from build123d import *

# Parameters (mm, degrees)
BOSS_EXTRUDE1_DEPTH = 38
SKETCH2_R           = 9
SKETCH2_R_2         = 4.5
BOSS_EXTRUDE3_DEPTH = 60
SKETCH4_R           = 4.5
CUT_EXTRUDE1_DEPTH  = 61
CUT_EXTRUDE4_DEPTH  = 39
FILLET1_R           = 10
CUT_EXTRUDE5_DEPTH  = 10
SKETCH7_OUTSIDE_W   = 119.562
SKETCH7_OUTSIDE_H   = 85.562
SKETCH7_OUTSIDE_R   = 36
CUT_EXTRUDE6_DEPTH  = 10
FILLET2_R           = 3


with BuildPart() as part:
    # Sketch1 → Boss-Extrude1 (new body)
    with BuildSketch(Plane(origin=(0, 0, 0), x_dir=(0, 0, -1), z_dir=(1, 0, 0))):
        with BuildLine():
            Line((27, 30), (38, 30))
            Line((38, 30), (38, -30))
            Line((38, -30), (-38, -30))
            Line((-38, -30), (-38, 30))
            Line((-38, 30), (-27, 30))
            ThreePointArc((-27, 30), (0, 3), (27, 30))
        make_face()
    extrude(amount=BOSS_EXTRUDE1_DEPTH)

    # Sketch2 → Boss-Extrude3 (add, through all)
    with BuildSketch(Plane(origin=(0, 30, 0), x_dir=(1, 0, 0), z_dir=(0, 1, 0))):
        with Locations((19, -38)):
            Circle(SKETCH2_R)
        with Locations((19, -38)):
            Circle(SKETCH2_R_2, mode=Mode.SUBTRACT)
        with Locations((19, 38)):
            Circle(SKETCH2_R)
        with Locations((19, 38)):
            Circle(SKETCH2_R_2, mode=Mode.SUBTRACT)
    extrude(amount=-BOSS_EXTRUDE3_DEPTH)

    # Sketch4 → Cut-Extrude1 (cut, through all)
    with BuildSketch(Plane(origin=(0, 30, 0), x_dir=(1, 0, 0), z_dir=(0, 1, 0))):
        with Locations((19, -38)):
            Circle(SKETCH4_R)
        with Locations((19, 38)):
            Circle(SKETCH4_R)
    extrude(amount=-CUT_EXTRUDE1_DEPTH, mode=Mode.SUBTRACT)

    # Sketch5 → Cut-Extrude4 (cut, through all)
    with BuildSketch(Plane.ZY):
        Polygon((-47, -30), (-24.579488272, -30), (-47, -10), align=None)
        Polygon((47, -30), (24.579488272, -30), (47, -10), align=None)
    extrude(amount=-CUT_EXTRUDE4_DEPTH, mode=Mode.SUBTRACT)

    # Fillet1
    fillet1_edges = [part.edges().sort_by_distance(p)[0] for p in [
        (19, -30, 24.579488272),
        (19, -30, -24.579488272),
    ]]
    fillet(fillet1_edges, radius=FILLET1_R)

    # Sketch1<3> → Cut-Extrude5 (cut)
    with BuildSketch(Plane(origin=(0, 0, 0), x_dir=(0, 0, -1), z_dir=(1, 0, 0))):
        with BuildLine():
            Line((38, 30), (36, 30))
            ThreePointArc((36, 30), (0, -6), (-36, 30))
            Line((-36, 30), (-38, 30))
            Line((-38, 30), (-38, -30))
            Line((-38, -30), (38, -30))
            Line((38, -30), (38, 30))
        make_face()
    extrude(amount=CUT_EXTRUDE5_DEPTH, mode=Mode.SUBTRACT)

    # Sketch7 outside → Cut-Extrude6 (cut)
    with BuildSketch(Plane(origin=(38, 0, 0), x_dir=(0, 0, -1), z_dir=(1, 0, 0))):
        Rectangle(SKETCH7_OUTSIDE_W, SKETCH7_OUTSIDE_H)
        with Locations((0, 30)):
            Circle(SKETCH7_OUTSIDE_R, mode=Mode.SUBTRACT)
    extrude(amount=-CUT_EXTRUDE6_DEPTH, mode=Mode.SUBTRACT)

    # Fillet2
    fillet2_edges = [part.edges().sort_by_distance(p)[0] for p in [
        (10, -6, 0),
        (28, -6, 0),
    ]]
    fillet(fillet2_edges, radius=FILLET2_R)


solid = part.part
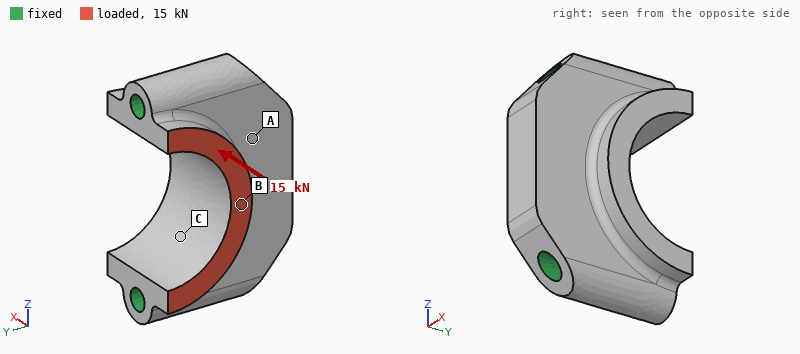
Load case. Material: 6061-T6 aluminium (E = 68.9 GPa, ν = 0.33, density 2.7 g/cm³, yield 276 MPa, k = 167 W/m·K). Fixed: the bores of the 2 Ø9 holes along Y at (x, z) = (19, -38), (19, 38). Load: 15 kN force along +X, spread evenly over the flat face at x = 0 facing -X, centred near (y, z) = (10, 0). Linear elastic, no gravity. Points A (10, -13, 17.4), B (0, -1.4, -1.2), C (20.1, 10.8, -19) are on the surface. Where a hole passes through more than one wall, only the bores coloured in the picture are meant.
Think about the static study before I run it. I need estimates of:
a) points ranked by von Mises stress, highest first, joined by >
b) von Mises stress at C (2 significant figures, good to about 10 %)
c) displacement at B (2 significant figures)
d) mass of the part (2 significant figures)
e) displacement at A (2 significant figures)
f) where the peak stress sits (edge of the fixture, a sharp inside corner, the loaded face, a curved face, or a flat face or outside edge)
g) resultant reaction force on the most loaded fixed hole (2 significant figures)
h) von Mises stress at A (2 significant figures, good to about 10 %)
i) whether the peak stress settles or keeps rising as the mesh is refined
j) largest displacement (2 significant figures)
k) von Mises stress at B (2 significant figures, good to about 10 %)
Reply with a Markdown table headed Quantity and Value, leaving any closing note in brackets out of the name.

| Quantity | Value |
|---|---|
| points ranked by von Mises stress, highest first, joined by > | B > C > A |
| von Mises stress at C | 12 MPa |
| displacement at B | 15 µm |
| mass of the part | 220 g |
| displacement at A | 7.7 µm |
| where the peak stress sits | edge of the fixture |
| resultant reaction force on the most loaded fixed hole | 7.5 kN |
| von Mises stress at A | 5.9 MPa |
| whether the peak stress settles or keeps rising as the mesh is refined | keeps rising |
| largest displacement | 15 µm |
| von Mises stress at B | 20 MPa |
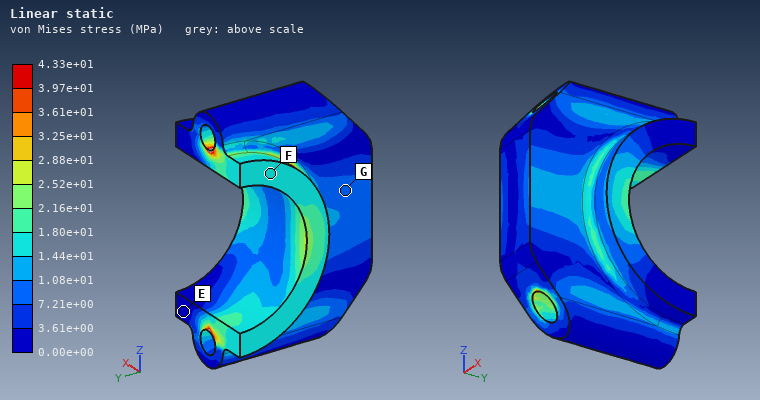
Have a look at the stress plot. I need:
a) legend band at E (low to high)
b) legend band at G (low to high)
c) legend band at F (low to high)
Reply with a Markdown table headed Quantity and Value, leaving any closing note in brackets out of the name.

| Quantity | Value |
|---|---|
| legend band at E | 0.00e+00 to 3.61e+00 MPa |
| legend band at G | 7.21e+00 to 1.08e+01 MPa |
| legend band at F | 1.44e+01 to 1.80e+01 MPa |
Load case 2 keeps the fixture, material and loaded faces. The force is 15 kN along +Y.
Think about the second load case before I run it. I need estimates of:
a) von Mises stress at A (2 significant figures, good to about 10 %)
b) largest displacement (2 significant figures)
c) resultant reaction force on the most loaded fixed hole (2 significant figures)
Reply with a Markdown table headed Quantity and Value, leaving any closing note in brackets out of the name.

| Quantity | Value |
|---|---|
| von Mises stress at A | 16 MPa |
| largest displacement | 41 µm |
| resultant reaction force on the most loaded fixed hole | 7.7 kN |
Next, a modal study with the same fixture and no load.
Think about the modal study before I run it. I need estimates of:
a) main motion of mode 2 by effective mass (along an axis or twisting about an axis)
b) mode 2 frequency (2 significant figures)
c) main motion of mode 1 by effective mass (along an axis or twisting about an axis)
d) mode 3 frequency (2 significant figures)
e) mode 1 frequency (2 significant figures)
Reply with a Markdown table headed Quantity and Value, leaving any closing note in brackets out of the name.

| Quantity | Value |
|---|---|
| main motion of mode 2 by effective mass | along Y |
| mode 2 frequency | 19 kHz |
| main motion of mode 1 by effective mass | along X |
| mode 3 frequency | 20 kHz |
| mode 1 frequency | 12 kHz |
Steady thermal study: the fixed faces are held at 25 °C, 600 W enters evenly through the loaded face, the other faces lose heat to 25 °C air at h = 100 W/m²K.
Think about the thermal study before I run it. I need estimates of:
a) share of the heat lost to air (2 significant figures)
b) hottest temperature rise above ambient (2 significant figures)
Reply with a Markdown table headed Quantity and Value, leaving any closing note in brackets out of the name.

| Quantity | Value |
|---|---|
| share of the heat lost to air | 4.5 % |
| hottest temperature rise above ambient | 84 K |
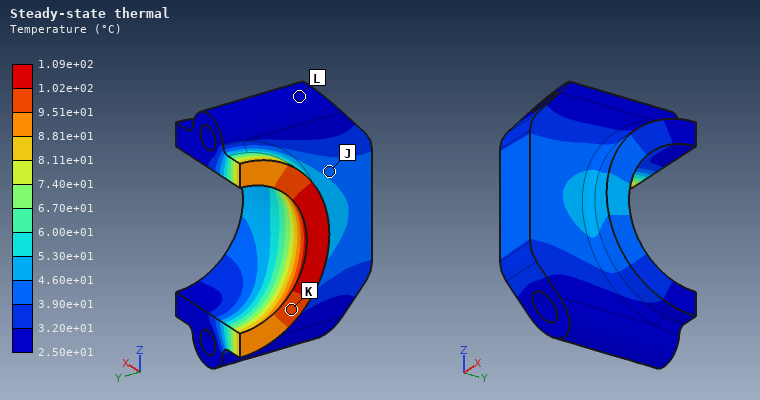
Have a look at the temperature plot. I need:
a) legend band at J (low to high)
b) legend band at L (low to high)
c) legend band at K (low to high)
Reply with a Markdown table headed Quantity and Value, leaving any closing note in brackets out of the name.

| Quantity | Value |
|---|---|
| legend band at J | 3.90e+01 to 4.60e+01 °C |
| legend band at L | 2.50e+01 to 3.20e+01 °C |
| legend band at K | 9.51e+01 to 1.02e+02 °C |
